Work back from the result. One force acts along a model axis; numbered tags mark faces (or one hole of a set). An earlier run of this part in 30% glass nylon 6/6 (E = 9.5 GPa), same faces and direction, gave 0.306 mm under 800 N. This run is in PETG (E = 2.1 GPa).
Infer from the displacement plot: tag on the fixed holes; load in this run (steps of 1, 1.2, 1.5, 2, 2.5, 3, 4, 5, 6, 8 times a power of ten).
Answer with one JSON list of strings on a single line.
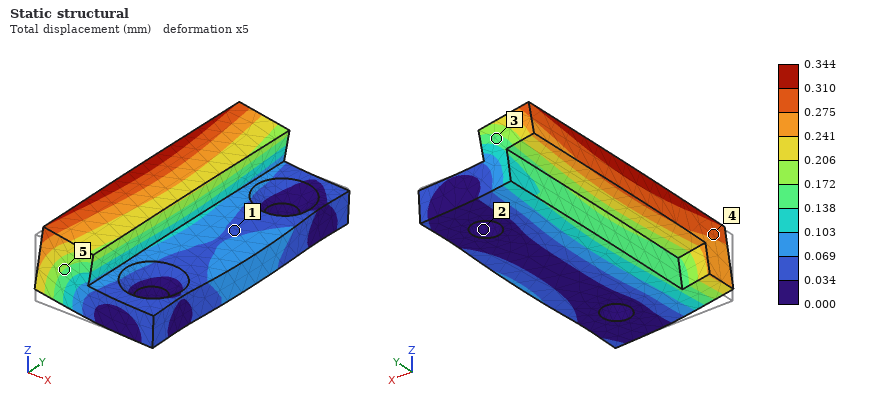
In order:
["2", "200 N"]
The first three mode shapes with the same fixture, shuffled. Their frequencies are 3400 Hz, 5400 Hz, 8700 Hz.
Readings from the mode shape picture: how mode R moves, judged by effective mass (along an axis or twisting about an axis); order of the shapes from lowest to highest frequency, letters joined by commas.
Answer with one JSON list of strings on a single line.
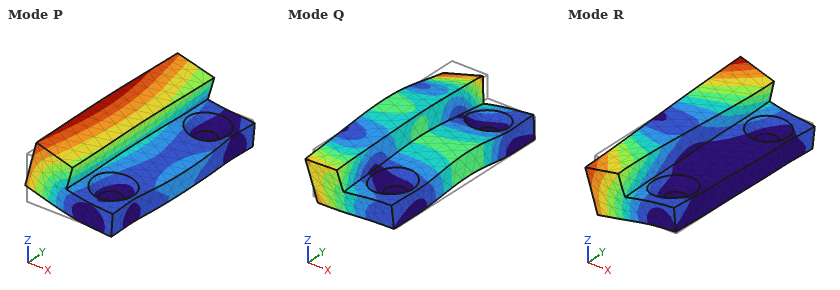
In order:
["twisting about X", "P, R, Q"]
